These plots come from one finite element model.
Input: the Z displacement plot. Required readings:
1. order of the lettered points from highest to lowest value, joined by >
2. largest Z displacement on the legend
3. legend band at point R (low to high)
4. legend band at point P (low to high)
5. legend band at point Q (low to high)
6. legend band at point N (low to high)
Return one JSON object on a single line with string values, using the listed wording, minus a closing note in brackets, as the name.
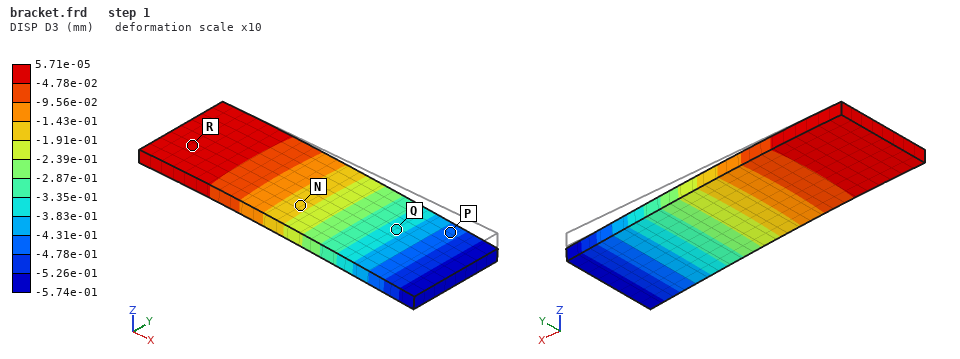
{"order of the lettered points from highest to lowest value, joined by >": "R > N > Q > P", "largest Z displacement on the legend": "5.71e-05 mm", "legend band at point R": "-4.78e-02 to 5.71e-05 mm", "legend band at point P": "-4.78e-01 to -4.31e-01 mm", "legend band at point Q": "-3.83e-01 to -3.35e-01 mm", "legend band at point N": "-1.91e-01 to -1.43e-01 mm"}
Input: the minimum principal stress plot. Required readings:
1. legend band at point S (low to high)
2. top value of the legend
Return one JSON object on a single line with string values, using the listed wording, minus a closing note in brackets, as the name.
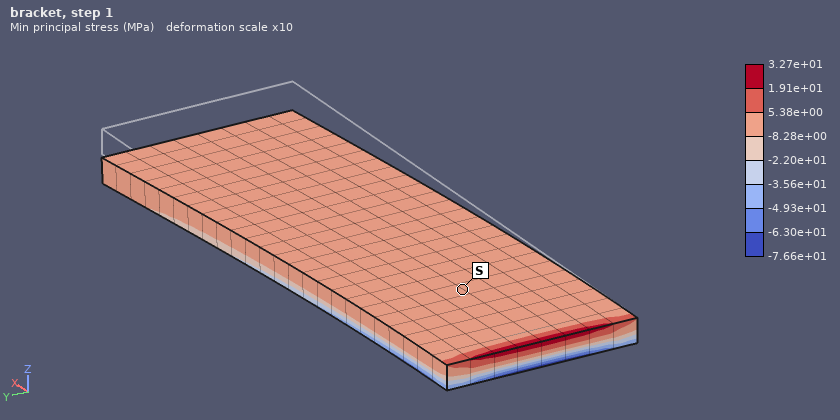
{"legend band at point S": "-8.28e+00 to 5.38e+00 MPa", "top value of the legend": "3.27e+01 MPa"}
